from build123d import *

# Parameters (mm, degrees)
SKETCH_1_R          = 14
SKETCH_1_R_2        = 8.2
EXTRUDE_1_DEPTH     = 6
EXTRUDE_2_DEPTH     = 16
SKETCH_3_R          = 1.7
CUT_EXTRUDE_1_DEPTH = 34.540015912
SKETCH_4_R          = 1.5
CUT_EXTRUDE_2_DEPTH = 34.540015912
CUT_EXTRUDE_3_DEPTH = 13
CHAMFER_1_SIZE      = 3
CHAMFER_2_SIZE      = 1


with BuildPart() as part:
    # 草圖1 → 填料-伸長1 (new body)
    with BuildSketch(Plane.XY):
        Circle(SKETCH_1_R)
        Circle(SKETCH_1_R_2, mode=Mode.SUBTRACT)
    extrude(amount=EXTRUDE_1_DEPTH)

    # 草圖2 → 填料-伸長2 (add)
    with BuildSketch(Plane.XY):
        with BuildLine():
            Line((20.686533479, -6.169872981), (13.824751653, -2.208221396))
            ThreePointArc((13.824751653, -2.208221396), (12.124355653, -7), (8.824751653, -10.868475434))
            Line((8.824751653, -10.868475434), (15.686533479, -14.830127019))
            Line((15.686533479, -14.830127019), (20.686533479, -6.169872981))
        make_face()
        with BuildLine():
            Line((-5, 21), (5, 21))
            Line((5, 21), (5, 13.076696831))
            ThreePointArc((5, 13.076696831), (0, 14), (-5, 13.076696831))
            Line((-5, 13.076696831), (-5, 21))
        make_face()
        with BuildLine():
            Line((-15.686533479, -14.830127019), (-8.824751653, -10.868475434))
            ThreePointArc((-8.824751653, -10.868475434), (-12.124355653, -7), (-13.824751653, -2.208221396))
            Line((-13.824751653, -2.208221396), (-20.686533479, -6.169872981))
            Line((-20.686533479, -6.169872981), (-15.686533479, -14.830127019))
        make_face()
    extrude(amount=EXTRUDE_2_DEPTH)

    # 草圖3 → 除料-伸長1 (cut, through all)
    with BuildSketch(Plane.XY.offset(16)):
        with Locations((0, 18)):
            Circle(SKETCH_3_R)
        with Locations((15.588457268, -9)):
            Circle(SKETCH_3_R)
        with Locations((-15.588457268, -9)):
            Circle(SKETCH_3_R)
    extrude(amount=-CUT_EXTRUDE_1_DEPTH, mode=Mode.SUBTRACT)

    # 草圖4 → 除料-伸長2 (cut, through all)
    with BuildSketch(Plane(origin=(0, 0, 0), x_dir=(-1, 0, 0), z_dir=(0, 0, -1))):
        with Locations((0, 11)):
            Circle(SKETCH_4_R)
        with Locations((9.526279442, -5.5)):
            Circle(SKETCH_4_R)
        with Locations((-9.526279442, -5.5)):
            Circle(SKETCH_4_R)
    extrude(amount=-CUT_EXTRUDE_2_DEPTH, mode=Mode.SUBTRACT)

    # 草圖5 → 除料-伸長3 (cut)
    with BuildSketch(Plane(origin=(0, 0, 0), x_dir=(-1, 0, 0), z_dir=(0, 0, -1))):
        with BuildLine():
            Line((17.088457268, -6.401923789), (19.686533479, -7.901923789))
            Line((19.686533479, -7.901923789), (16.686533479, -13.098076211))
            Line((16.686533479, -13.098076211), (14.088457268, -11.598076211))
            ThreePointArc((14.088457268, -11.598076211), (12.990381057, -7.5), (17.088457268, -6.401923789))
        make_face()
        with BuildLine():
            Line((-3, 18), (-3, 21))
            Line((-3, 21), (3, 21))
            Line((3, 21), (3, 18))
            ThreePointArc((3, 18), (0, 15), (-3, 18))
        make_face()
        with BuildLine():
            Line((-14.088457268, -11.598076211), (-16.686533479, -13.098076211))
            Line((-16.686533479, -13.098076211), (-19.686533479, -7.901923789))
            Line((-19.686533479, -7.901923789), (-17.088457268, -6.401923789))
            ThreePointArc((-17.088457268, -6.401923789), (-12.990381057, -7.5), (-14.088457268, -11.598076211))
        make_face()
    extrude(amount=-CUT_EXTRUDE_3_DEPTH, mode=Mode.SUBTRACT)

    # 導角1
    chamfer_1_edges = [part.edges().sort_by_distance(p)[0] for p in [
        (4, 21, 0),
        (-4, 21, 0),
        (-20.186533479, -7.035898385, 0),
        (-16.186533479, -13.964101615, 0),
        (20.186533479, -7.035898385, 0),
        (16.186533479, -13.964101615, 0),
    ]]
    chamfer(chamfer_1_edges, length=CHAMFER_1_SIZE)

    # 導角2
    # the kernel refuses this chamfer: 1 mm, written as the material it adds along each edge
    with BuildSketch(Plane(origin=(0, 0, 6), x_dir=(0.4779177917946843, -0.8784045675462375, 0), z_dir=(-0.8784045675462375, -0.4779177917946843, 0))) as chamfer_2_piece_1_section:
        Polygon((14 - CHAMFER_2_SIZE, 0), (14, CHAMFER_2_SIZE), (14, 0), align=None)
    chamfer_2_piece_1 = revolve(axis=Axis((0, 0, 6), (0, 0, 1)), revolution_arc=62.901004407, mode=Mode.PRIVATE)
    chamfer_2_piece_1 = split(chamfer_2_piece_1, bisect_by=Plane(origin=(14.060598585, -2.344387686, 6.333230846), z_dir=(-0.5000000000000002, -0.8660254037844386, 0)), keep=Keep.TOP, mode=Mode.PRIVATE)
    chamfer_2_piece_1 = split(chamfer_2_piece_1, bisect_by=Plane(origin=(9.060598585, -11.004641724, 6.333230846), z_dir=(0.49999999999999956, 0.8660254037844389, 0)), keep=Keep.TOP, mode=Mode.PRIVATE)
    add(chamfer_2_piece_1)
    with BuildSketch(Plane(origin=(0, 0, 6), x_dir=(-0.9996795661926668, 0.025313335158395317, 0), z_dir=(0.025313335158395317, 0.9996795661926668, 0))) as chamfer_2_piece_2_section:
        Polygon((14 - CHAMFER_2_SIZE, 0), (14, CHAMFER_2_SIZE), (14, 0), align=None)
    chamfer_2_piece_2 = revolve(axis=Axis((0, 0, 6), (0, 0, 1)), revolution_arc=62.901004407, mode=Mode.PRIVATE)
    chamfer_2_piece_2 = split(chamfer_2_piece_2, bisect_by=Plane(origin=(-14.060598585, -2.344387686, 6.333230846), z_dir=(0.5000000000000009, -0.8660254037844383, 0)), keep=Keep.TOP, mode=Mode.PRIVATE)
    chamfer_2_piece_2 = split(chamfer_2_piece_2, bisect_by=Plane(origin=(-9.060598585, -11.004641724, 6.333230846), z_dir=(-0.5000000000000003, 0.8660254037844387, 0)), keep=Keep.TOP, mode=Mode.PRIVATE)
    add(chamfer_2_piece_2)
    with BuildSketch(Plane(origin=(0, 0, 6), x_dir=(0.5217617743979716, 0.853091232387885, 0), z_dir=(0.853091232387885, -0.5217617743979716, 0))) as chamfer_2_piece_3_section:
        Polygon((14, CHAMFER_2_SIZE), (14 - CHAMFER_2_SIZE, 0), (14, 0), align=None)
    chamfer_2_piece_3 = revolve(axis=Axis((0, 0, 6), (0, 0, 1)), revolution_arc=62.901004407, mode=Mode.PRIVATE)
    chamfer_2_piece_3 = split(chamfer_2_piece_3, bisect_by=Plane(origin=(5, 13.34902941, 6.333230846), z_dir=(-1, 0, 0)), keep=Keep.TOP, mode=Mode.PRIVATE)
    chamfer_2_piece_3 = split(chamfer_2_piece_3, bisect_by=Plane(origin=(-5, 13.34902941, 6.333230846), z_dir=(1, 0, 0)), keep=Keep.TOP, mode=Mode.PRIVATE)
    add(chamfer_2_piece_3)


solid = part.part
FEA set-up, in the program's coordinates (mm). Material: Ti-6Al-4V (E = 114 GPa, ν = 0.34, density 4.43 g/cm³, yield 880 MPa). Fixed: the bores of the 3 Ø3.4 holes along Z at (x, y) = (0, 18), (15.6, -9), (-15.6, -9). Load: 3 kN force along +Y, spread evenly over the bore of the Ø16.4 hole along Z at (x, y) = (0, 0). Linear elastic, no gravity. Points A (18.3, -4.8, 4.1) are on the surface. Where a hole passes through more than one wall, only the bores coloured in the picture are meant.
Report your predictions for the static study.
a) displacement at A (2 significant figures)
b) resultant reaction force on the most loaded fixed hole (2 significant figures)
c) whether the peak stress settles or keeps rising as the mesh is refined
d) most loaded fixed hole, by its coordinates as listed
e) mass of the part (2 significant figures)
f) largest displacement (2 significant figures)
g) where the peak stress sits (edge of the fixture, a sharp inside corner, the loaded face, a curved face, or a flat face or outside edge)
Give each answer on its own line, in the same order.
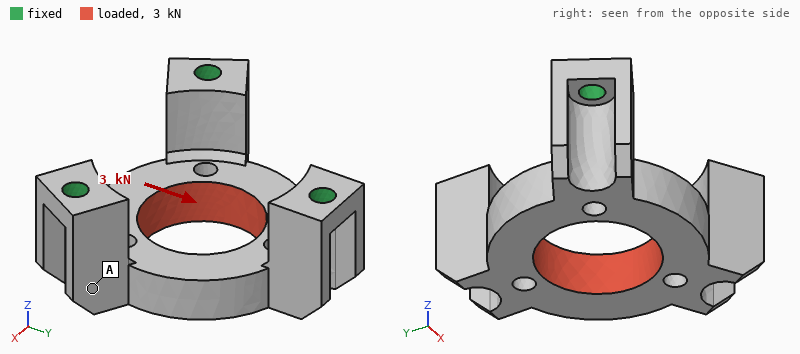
29 µm
1.4 kN
keeps rising
(0, 18)
20 g
47 µm
edge of the fixture
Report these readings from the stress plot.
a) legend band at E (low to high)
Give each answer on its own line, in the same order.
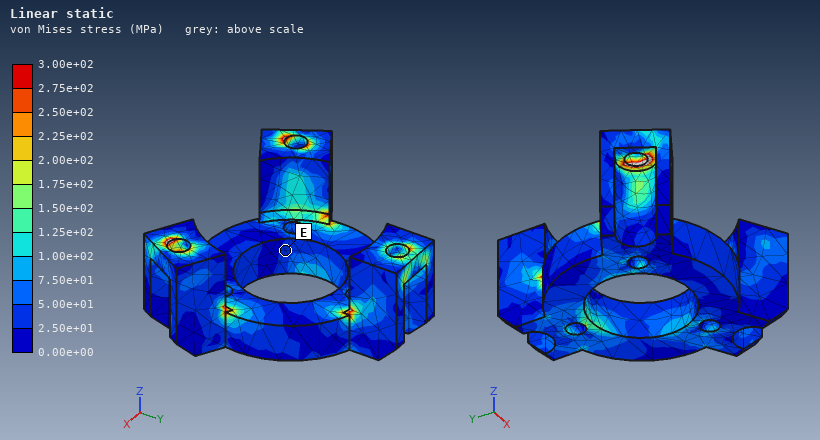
2.50e+01 to 5.00e+01 MPa
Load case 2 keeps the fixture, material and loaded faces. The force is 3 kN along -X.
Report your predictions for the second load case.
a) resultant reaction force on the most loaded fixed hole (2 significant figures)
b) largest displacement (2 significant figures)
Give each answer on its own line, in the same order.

1.3 kN
44 µm
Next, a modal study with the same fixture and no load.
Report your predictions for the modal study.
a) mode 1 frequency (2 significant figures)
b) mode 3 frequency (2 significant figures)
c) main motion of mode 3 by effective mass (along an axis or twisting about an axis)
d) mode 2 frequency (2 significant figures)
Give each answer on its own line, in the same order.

12 kHz
15 kHz
twisting about Z
12 kHz
